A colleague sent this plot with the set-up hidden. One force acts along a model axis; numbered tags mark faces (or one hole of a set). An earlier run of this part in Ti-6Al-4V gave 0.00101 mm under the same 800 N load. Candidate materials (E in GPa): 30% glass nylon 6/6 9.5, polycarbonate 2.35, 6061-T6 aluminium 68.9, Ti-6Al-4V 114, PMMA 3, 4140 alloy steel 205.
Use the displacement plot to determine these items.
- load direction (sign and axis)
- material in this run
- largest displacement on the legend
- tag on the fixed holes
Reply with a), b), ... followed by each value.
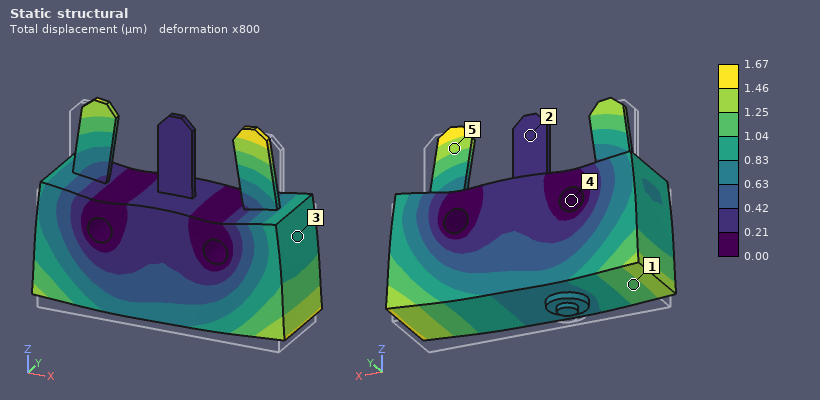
a) +Z
b) 6061-T6 aluminium
c) 1.67 µm
d) 4
